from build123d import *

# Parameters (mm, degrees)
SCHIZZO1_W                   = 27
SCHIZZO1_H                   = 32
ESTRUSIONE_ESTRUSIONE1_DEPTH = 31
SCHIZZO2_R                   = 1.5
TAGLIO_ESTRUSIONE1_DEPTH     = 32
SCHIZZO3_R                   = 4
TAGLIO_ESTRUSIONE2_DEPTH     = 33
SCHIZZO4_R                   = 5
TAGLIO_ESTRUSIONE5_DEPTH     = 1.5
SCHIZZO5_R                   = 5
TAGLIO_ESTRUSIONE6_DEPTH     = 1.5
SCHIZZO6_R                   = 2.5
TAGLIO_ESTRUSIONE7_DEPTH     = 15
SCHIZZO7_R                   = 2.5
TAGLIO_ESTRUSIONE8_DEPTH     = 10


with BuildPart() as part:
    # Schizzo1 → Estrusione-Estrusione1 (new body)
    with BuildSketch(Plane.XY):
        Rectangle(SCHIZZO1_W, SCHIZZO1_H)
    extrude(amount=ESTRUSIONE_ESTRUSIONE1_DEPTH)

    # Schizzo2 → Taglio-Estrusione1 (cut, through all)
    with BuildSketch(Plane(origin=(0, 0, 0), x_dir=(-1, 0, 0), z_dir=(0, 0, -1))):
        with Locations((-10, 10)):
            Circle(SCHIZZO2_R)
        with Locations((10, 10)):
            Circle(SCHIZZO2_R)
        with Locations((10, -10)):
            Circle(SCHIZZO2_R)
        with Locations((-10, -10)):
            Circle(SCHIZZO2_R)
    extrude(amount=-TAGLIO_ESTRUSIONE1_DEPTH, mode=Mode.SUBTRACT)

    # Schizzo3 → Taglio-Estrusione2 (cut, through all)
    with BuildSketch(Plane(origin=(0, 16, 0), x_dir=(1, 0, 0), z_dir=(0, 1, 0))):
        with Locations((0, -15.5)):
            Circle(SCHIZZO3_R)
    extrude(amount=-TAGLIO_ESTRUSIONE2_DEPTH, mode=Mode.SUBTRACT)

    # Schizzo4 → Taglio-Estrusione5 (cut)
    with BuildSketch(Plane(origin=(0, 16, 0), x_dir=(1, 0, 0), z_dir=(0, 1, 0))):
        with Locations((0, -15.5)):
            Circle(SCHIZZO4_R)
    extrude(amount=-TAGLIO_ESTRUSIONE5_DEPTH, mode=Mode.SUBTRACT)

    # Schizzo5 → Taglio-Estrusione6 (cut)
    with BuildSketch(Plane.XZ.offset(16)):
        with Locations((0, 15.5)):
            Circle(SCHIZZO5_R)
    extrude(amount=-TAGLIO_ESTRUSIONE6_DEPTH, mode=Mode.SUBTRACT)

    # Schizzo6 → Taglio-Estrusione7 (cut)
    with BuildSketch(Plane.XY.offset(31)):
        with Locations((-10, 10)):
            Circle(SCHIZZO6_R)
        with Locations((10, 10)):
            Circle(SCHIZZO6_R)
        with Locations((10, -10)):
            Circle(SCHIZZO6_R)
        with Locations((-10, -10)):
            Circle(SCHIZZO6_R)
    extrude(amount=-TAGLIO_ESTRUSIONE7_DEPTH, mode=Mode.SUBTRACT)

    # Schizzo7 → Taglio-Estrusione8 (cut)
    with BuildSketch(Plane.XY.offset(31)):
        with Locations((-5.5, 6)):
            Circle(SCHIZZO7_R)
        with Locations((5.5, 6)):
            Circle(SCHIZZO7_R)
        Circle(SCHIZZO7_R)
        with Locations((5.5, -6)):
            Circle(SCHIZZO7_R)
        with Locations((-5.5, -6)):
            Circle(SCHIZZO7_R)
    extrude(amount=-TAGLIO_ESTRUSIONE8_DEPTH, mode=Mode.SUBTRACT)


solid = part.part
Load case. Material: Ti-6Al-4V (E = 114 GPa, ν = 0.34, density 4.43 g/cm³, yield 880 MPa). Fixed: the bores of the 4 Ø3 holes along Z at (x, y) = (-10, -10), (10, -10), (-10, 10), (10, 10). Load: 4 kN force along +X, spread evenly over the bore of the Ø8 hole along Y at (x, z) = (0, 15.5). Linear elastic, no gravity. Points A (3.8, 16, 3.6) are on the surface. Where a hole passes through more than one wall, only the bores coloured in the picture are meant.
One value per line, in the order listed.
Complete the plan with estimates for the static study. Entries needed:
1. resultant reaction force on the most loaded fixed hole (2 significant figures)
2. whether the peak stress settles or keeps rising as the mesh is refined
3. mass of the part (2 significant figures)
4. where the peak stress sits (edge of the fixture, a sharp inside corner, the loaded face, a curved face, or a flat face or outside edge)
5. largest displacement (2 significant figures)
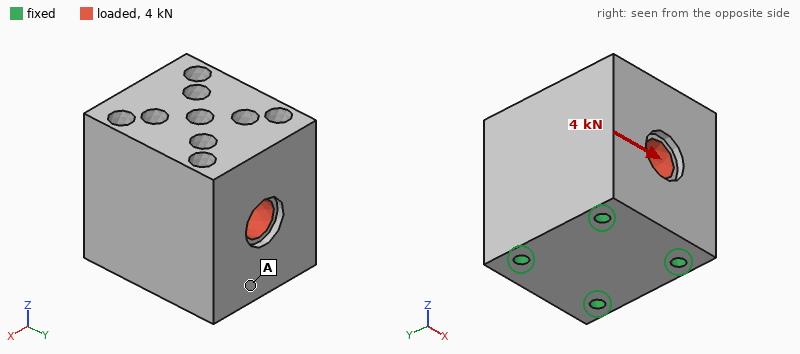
1.1 kN
keeps rising
100 g
edge of the fixture
1.5 µm
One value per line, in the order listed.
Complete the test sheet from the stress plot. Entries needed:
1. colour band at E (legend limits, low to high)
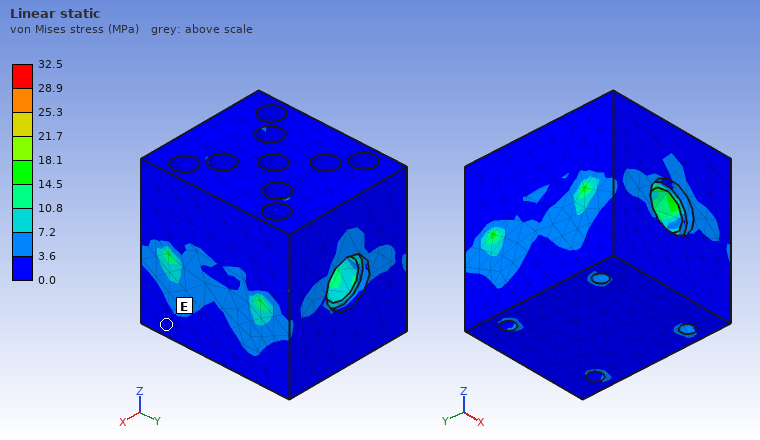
0.0 to 3.6 MPa
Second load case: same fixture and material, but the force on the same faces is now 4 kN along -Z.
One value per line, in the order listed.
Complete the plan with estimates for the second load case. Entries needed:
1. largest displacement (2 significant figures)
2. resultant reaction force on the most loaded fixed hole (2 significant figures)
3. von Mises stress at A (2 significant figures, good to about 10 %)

1.4 µm
1.0 kN
2.8 MPa
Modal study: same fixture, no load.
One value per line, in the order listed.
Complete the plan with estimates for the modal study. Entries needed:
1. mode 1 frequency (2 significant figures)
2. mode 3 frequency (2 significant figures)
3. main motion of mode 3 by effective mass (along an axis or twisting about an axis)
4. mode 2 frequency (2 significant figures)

26 kHz
34 kHz
twisting about Z
26 kHz
